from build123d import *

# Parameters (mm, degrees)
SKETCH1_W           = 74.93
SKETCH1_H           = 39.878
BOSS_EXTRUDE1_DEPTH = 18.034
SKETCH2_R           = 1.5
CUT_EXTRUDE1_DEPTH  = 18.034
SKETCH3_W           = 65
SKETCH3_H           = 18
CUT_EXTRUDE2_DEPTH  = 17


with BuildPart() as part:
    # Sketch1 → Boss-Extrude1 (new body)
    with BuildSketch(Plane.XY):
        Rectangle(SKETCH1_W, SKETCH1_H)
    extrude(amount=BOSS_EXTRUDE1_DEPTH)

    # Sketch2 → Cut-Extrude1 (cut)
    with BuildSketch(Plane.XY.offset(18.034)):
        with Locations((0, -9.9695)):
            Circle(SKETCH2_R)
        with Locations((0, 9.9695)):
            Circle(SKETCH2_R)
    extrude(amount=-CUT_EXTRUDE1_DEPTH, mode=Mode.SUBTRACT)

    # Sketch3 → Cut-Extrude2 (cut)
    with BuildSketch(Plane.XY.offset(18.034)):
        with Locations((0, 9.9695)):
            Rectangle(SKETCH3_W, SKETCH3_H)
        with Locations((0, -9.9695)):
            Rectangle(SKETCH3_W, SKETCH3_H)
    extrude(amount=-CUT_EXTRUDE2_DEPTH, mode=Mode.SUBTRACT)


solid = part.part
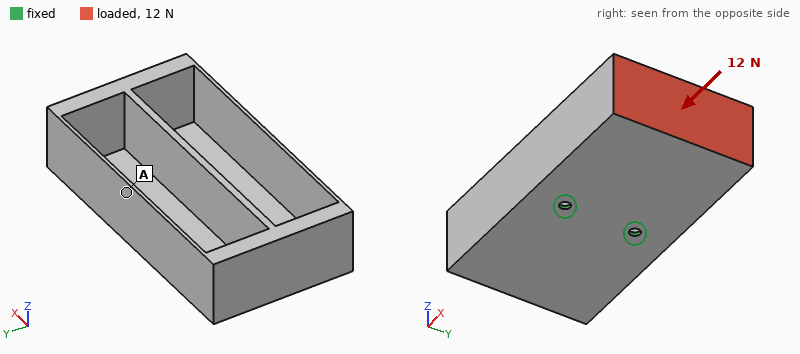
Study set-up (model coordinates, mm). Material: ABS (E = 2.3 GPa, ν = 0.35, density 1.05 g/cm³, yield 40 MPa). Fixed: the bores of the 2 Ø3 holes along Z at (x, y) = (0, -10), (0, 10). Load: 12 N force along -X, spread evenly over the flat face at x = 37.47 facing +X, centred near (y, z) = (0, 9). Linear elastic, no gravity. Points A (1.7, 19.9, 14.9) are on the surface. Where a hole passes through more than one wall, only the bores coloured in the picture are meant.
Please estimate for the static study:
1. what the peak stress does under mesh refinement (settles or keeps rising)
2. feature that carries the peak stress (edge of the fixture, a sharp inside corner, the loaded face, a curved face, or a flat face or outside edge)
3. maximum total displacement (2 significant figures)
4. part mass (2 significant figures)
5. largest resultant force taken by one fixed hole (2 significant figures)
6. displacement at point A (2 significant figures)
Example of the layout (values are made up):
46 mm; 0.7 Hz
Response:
keeps rising; edge of the fixture; 0.97 mm; 15 g; 6.0 N; 0.34 mm
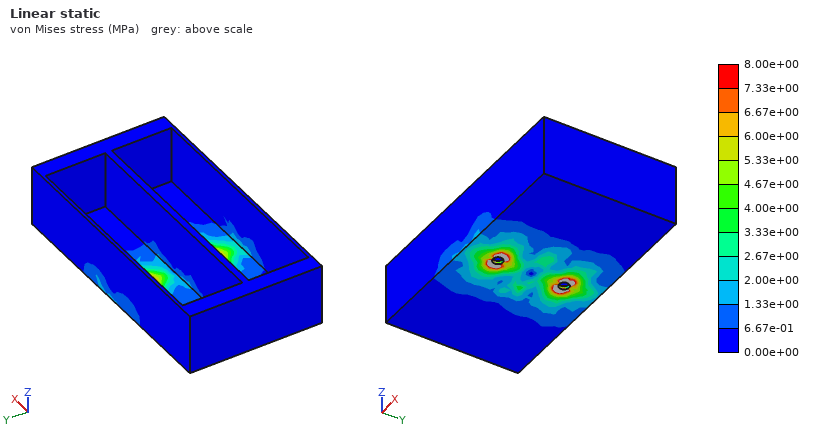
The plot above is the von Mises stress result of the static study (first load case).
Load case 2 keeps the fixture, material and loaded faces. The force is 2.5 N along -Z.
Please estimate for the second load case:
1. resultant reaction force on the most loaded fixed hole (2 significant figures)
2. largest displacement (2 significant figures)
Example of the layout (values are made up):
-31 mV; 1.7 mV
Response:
1.3 N; 0.90 mm
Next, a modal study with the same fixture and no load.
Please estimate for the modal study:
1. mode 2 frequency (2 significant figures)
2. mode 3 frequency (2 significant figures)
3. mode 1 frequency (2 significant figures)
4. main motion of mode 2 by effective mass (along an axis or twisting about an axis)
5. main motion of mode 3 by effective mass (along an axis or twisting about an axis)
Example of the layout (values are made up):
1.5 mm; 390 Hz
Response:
350 Hz; 550 Hz; 92 Hz; along Y; along Z
